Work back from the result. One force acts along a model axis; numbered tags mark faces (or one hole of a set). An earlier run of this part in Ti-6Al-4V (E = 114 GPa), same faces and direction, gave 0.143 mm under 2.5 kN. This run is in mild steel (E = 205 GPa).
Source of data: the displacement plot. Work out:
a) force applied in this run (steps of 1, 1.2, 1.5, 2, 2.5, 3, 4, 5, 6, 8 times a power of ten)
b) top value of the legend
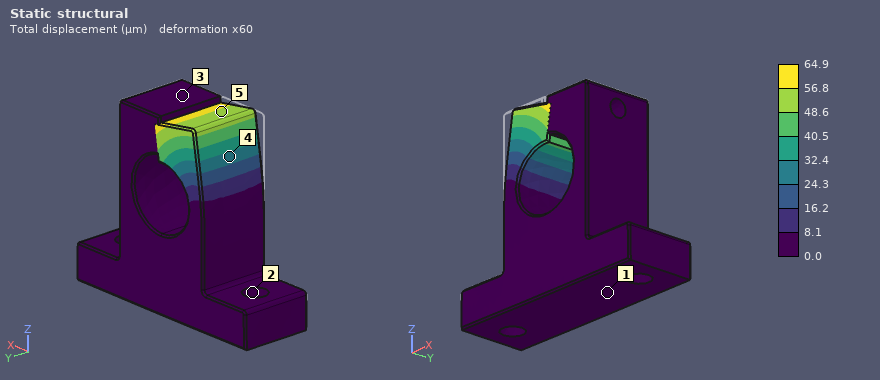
2 kN
64.9 µm
